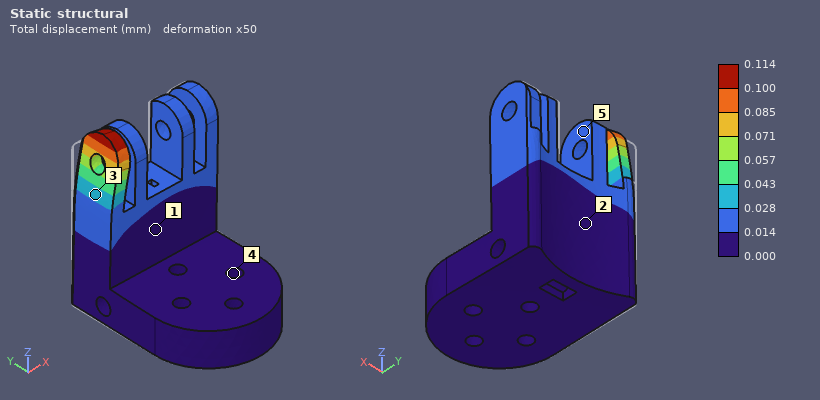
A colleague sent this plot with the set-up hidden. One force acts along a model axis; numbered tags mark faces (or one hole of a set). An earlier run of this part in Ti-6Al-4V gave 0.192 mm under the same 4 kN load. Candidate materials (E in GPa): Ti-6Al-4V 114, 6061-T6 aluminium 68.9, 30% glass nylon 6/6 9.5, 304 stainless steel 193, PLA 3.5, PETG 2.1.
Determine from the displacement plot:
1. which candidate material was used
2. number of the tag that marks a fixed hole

304 stainless steel
4
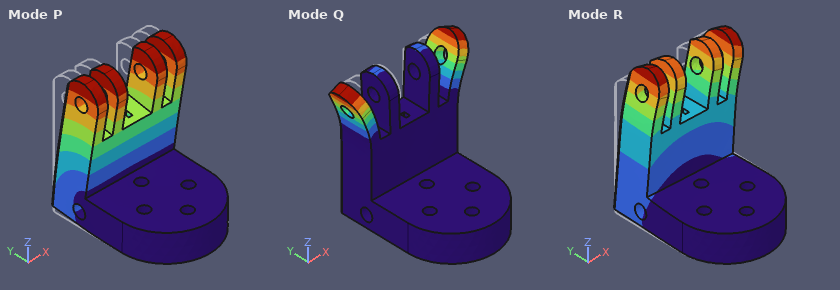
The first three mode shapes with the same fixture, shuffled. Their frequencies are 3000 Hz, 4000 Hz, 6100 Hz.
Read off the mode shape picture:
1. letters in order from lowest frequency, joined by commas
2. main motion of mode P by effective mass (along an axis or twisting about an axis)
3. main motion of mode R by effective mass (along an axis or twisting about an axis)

P, R, Q
along Y
along X
